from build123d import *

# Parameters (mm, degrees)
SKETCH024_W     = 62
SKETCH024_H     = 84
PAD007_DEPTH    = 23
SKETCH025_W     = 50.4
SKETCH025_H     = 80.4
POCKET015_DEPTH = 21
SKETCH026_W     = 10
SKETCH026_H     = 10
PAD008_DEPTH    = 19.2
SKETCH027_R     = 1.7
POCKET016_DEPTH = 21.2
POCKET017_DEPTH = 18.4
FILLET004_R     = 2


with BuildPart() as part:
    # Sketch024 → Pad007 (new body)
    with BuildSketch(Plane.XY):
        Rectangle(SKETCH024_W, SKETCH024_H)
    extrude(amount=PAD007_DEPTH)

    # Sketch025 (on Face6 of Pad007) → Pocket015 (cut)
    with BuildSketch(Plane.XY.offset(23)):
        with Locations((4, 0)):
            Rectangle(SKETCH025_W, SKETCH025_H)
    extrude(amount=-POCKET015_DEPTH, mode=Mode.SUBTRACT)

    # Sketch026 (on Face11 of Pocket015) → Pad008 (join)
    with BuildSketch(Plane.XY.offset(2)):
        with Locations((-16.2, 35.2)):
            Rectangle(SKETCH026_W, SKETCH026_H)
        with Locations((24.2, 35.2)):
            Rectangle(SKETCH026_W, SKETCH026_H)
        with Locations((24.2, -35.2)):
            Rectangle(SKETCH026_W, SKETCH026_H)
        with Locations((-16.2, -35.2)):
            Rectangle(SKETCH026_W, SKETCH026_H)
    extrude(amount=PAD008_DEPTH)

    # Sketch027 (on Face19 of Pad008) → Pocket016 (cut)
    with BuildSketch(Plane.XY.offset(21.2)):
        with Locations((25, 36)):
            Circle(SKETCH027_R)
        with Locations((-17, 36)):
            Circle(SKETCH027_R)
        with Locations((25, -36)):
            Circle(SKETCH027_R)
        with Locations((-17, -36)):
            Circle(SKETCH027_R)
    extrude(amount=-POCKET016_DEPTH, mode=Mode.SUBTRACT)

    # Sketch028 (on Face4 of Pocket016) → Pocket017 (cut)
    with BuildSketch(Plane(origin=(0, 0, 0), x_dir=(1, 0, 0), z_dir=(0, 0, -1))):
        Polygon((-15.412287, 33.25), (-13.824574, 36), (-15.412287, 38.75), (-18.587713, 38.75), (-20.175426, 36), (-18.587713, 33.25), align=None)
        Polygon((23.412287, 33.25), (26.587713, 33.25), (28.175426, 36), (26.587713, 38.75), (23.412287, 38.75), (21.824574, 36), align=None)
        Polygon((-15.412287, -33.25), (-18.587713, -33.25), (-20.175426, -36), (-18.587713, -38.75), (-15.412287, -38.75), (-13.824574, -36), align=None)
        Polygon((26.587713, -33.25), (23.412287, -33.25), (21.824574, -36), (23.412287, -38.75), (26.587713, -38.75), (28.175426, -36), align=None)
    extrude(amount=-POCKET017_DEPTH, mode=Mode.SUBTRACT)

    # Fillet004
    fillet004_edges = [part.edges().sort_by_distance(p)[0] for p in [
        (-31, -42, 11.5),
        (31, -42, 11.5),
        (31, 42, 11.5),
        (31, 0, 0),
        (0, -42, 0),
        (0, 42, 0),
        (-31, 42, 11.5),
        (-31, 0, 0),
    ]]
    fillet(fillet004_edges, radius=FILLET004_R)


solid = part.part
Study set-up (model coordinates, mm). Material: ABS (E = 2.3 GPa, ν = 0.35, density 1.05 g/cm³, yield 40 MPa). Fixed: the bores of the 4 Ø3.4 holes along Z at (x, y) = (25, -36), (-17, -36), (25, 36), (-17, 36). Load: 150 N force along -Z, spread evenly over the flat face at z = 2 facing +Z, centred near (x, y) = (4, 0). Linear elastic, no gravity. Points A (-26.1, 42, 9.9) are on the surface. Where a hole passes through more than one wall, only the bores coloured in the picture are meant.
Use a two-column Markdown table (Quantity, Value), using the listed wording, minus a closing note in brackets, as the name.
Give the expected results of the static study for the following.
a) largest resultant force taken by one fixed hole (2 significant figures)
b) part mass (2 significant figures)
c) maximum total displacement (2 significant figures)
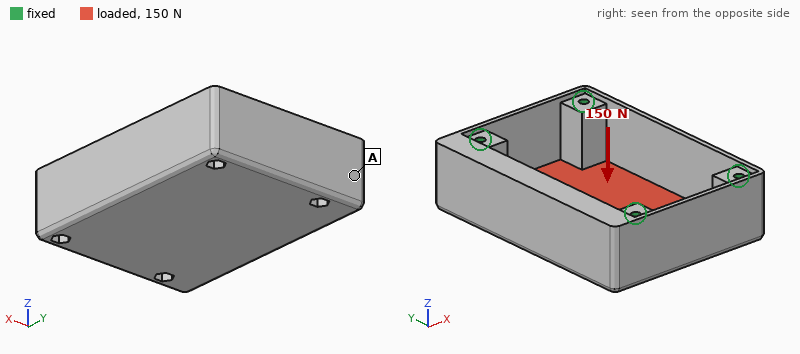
| Quantity | Value |
|---|---|
| largest resultant force taken by one fixed hole | 43 N |
| part mass | 42 g |
| maximum total displacement | 0.50 mm |
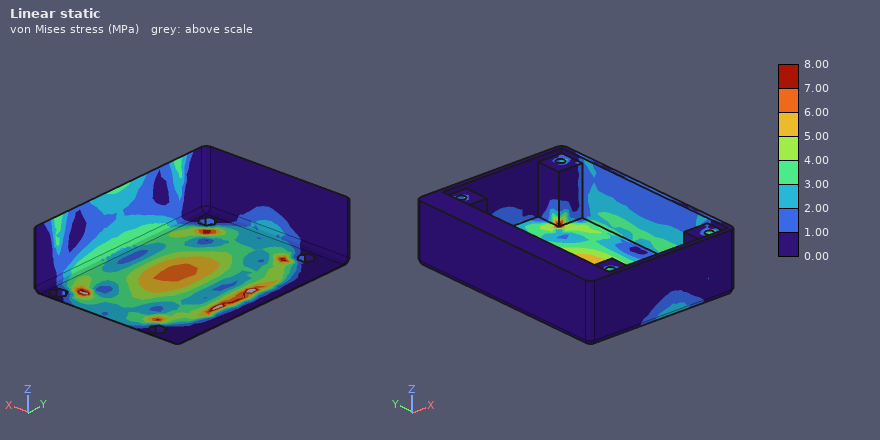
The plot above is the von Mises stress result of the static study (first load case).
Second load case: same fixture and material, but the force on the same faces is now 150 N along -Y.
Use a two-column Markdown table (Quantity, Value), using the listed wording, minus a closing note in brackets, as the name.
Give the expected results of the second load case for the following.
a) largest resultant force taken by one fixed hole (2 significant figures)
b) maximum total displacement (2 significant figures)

| Quantity | Value |
|---|---|
| largest resultant force taken by one fixed hole | 47 N |
| maximum total displacement | 28 µm |
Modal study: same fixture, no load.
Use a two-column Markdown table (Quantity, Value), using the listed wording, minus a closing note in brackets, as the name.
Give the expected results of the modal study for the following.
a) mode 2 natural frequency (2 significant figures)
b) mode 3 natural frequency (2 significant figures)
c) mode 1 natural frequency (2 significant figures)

| Quantity | Value |
|---|---|
| mode 2 natural frequency | 1400 Hz |
| mode 3 natural frequency | 1900 Hz |
| mode 1 natural frequency | 1100 Hz |
